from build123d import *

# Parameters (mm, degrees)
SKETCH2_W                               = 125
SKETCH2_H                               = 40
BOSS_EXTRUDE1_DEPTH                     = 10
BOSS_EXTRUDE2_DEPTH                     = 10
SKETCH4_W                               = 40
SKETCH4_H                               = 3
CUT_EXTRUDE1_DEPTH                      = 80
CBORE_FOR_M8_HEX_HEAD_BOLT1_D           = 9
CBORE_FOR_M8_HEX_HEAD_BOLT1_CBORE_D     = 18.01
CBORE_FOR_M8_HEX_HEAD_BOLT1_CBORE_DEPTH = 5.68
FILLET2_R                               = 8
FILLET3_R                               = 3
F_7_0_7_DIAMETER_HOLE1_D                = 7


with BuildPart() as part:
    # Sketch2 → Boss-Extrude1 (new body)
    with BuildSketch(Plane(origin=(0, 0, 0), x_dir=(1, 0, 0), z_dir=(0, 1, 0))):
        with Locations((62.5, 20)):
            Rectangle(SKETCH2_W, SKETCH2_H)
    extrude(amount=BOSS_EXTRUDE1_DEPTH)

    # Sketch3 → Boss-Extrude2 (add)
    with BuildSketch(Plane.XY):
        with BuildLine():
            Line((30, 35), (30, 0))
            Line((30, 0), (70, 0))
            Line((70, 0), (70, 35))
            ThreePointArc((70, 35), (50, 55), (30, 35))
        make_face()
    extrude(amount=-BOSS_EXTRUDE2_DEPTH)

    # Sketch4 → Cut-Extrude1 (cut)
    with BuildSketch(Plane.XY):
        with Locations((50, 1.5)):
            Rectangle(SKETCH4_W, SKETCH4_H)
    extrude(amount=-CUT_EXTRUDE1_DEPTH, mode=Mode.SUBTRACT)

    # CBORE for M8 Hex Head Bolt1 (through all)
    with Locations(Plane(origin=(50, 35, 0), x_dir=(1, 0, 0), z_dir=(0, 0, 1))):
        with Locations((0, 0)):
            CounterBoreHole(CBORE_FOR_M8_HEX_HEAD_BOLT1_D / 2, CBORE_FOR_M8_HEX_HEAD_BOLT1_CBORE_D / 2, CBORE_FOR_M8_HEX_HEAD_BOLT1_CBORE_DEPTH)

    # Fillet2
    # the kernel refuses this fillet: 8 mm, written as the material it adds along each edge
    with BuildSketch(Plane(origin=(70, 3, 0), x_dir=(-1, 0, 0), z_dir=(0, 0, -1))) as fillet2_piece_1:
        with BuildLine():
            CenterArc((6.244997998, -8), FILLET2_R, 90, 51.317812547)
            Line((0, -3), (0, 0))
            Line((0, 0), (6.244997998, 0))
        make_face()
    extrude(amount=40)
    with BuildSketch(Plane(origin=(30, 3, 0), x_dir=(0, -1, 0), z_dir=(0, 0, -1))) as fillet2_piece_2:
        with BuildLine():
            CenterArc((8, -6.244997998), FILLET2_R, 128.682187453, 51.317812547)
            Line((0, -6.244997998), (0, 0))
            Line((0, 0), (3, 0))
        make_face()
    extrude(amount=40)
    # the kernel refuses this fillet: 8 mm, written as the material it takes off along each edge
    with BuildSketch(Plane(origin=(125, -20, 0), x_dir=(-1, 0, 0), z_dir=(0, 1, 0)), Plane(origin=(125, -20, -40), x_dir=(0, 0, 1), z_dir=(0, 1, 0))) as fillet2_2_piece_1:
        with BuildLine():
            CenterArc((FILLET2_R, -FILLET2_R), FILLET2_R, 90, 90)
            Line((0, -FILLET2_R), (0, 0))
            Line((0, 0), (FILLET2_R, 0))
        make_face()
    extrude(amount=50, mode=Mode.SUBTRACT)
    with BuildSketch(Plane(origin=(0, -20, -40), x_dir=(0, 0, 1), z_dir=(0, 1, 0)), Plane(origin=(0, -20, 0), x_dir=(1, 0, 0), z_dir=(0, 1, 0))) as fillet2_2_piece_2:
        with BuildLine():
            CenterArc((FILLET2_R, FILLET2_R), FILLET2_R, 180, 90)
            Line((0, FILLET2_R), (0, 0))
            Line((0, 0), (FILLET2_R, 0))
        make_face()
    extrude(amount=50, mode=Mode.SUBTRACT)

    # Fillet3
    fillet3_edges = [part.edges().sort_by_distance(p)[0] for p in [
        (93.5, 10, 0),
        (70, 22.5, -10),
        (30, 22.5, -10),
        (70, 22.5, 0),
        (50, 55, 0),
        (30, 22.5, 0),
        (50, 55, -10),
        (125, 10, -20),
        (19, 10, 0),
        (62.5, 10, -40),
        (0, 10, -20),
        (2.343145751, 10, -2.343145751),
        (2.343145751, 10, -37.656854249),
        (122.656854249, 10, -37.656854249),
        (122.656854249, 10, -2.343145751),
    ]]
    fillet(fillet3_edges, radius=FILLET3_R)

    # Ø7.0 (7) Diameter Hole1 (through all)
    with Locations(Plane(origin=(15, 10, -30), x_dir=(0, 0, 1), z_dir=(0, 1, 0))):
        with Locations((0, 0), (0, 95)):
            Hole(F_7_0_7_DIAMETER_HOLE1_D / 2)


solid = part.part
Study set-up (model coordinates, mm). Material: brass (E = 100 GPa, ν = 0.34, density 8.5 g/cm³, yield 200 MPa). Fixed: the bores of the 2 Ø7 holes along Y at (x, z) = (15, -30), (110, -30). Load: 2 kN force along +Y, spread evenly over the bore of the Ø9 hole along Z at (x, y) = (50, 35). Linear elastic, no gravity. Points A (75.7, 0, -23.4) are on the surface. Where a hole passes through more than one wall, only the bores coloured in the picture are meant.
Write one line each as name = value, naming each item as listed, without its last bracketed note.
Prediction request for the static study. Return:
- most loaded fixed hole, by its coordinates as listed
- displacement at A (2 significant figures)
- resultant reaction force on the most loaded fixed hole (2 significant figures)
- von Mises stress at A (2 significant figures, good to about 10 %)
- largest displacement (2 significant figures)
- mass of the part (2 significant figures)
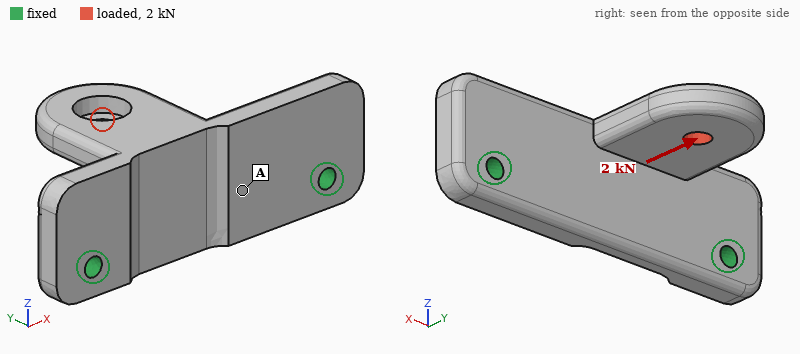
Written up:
most loaded fixed hole, by its coordinates as listed = (15, -30)
displacement at A = 25 µm
resultant reaction force on the most loaded fixed hole = 1.4 kN
von Mises stress at A = 15 MPa
largest displacement = 83 µm
mass of the part = 490 g
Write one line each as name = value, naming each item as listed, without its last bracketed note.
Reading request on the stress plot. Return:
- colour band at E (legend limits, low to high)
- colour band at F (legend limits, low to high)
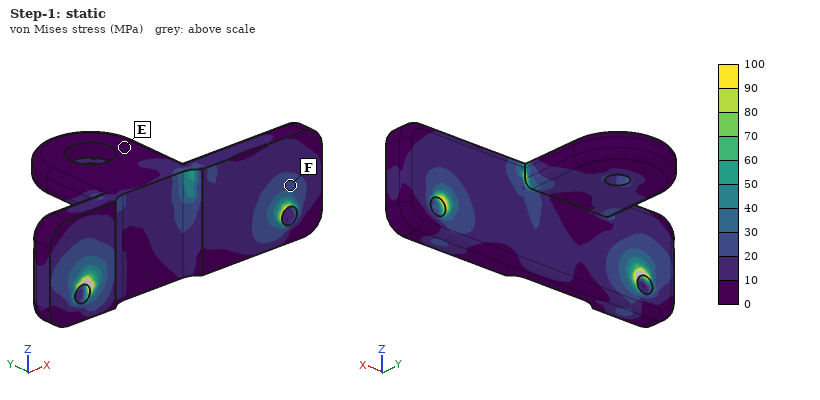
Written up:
colour band at E = 0 to 10 MPa
colour band at F = 20 to 30 MPa
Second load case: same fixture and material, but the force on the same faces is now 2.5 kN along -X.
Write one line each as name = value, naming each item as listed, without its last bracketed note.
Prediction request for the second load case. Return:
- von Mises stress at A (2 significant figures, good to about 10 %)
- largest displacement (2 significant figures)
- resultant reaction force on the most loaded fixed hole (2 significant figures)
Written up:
von Mises stress at A = 17 MPa
largest displacement = 0.10 mm
resultant reaction force on the most loaded fixed hole = 1.8 kN
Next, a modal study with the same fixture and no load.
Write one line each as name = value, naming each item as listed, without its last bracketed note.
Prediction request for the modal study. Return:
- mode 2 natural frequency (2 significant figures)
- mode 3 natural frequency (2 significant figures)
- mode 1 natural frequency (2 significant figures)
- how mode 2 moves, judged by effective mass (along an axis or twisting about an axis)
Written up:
mode 2 natural frequency = 2300 Hz
mode 3 natural frequency = 3200 Hz
mode 1 natural frequency = 1400 Hz
how mode 2 moves, judged by effective mass = along Y
